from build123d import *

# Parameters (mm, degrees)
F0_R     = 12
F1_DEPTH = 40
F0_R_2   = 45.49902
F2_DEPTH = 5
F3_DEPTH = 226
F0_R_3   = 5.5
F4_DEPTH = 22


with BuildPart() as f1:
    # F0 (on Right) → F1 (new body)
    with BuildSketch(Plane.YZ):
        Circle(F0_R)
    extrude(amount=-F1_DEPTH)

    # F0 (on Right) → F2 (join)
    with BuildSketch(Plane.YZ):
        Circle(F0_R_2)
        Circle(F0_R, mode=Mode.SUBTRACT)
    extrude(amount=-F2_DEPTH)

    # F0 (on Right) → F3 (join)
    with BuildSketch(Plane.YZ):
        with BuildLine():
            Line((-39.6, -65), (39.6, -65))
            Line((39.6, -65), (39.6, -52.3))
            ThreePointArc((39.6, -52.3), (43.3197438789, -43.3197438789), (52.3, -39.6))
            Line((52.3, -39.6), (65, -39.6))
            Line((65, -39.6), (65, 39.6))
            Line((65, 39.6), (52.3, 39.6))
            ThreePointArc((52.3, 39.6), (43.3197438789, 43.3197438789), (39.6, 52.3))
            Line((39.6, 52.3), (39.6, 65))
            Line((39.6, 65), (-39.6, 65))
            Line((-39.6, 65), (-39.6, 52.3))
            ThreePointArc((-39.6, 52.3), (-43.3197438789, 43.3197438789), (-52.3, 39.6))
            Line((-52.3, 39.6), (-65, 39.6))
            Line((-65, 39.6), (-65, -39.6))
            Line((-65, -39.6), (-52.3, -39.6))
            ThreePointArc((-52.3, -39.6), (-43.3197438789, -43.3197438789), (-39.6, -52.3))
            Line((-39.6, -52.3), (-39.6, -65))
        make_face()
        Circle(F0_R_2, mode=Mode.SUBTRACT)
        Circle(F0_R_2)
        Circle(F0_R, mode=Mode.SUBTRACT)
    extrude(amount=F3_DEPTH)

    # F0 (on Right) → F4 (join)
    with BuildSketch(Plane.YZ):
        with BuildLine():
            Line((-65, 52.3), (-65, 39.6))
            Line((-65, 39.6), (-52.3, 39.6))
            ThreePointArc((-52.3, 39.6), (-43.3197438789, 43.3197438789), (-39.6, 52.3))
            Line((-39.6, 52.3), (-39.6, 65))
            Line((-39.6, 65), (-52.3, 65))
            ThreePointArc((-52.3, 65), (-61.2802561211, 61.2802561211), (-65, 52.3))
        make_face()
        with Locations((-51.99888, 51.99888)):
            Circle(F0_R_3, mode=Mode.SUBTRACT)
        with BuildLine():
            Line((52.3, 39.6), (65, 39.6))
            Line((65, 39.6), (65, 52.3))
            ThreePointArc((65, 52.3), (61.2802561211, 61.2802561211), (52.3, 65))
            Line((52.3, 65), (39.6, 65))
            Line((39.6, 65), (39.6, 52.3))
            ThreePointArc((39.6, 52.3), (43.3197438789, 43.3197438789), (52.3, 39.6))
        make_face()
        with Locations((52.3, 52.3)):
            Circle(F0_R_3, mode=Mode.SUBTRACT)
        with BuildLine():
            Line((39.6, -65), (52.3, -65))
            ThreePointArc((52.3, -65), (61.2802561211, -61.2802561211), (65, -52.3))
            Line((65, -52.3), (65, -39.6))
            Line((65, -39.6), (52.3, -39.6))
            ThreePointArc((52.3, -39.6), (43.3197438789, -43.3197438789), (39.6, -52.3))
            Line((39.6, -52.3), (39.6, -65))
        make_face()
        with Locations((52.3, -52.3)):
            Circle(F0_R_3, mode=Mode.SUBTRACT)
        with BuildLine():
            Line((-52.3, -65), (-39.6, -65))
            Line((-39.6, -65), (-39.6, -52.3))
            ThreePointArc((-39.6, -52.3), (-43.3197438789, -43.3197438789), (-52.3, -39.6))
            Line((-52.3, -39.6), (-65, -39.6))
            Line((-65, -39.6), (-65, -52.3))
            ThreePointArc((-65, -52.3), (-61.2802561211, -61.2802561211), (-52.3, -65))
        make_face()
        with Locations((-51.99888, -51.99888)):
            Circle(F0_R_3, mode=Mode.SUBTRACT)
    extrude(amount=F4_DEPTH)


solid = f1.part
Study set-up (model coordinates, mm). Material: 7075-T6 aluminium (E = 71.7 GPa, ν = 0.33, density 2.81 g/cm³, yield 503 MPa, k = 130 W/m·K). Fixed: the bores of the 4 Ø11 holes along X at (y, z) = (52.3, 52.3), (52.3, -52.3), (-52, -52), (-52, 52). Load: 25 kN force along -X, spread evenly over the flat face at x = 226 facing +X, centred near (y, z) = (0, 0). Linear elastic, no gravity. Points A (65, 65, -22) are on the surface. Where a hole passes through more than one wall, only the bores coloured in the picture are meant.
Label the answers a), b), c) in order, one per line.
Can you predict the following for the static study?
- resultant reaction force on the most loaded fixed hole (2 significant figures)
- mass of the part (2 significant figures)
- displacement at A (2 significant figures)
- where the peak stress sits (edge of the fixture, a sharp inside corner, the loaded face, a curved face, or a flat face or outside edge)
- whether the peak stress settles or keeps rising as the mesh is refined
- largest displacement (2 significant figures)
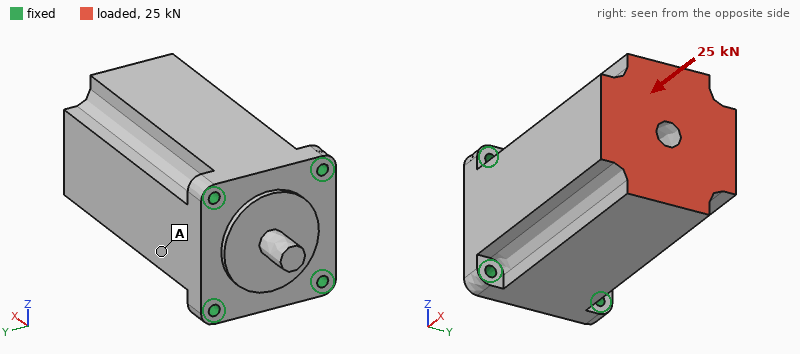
a) 6.5 kN
b) 9.1 kg
c) 7.1 µm
d) edge of the fixture
e) keeps rising
f) 11 µm
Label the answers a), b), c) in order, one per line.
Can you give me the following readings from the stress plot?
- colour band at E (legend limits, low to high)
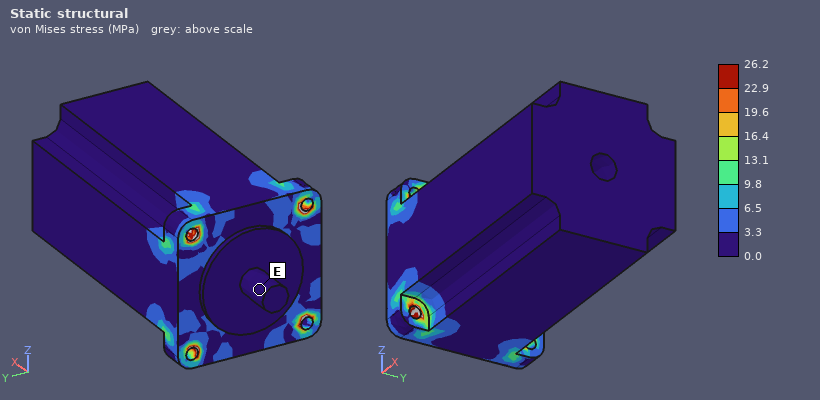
a) 0.0 to 3.3 MPa
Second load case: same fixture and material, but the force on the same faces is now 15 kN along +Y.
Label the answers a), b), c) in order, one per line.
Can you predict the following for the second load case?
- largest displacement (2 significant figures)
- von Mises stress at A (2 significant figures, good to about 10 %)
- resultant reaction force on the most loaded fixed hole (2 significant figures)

a) 0.12 mm
b) 9.2 MPa
c) 17 kN
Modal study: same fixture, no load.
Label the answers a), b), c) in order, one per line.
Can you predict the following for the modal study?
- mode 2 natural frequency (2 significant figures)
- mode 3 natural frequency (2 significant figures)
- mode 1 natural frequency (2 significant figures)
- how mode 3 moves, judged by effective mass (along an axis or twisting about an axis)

a) 1100 Hz
b) 3100 Hz
c) 1100 Hz
d) along X
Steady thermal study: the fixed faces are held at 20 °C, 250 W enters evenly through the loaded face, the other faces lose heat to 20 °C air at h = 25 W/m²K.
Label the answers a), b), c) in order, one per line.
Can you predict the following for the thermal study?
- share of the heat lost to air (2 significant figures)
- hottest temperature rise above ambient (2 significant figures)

a) 25 %
b) 32 K
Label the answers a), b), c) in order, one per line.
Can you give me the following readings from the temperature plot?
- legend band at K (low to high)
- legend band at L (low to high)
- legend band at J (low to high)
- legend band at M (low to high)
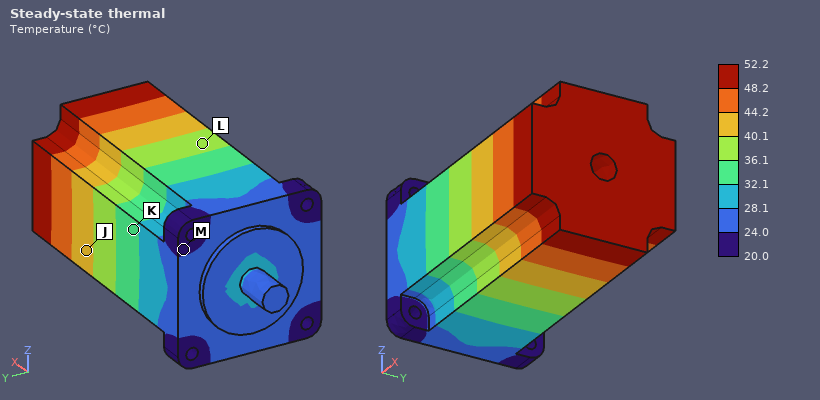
a) 32.1 to 36.1 °C
b) 36.1 to 40.1 °C
c) 40.1 to 44.2 °C
d) 20.0 to 24.0 °C
